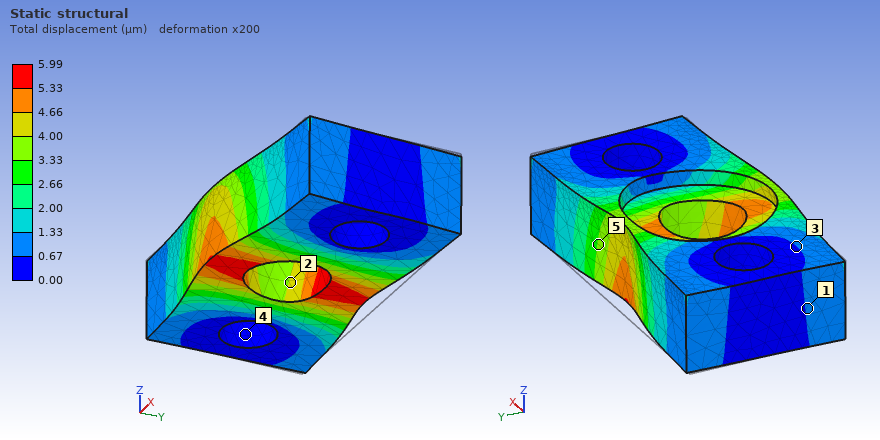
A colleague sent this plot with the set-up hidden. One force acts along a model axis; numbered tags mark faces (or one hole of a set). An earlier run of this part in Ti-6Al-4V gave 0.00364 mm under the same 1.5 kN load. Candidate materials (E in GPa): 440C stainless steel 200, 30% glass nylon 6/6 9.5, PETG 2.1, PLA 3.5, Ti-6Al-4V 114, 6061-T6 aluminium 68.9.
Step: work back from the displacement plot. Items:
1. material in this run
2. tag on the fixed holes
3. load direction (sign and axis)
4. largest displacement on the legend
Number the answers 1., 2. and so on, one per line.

1. 6061-T6 aluminium
2. 4
3. -Y
4. 5.99 µm
